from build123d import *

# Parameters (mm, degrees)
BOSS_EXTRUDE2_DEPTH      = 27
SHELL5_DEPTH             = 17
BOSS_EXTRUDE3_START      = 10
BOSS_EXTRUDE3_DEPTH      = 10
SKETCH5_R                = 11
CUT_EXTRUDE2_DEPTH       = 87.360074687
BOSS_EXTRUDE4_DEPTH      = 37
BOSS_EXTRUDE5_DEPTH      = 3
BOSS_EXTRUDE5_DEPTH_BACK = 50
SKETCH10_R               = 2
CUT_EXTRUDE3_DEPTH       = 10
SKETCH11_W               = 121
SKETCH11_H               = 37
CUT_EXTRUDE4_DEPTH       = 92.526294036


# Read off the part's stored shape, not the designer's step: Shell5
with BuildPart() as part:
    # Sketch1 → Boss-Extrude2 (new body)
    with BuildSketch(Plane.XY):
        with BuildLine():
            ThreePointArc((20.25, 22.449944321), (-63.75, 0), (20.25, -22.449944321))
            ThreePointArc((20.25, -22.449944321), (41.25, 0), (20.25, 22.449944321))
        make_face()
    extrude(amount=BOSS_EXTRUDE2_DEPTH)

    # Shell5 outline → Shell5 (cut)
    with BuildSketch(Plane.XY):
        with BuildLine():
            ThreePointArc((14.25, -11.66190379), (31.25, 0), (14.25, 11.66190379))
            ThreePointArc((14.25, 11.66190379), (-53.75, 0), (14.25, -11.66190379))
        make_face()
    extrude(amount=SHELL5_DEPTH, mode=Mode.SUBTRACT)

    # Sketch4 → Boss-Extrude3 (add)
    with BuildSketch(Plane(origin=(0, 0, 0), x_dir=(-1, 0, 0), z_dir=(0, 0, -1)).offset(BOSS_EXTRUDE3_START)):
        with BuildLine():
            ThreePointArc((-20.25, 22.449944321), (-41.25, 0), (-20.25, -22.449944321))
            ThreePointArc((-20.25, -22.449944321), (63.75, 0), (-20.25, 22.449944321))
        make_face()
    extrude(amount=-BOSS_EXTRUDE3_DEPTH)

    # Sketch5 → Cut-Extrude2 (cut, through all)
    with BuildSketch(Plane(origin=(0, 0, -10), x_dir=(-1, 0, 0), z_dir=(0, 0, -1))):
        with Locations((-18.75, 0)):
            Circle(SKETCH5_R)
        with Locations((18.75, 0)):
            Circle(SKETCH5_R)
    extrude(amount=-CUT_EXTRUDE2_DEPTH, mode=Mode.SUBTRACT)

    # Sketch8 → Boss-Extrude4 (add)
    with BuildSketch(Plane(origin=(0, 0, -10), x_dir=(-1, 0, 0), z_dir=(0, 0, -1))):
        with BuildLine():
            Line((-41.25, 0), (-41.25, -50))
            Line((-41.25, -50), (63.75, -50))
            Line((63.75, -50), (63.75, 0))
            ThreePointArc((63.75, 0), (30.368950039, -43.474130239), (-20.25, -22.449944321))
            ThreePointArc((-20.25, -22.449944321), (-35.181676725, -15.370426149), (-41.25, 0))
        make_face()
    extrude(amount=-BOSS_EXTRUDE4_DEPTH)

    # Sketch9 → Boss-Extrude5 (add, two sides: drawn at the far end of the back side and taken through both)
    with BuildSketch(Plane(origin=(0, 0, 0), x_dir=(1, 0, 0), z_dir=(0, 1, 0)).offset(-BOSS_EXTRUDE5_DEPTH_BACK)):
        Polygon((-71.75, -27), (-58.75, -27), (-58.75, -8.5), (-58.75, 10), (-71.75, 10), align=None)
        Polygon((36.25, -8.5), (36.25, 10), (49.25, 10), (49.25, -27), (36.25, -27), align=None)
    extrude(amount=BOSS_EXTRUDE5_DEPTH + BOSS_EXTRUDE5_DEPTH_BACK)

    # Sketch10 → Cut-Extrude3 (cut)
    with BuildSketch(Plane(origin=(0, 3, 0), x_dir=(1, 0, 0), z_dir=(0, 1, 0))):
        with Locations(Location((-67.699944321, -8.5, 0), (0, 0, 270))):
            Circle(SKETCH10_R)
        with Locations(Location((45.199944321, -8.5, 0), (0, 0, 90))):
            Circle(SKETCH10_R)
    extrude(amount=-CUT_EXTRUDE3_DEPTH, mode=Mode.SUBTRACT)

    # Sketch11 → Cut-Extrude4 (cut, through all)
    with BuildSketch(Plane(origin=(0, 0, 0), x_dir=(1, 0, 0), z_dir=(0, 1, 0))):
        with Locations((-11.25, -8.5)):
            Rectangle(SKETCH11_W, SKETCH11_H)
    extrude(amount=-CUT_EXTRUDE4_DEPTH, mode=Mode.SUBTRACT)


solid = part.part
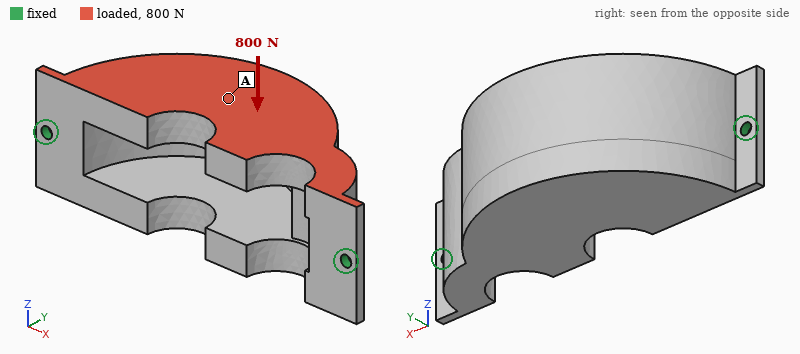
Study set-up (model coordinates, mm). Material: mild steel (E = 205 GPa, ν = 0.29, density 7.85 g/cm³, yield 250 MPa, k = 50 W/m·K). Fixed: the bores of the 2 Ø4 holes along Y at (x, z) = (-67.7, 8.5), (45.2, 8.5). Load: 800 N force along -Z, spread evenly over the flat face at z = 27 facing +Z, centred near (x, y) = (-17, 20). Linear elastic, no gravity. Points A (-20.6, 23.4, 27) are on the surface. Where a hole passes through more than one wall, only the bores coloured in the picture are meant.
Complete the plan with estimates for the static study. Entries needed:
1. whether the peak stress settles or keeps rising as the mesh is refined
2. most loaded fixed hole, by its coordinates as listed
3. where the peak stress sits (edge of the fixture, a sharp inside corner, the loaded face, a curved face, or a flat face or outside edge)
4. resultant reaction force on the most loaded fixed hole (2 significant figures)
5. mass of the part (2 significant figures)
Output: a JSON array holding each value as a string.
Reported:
["keeps rising", "(-67.7, 8.5)", "edge of the fixture", "430 N", "680 g"]
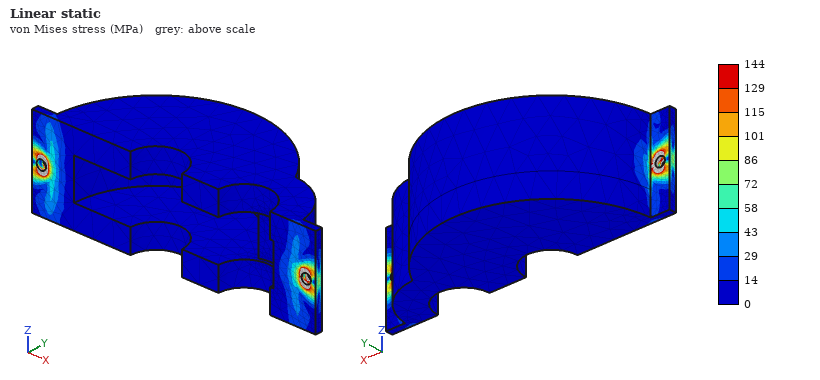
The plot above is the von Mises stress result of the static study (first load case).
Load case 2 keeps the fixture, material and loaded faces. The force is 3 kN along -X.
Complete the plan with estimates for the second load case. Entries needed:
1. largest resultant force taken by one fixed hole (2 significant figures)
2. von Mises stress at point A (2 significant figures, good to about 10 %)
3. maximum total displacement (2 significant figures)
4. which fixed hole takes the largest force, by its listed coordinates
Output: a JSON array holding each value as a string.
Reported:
["1.9 kN", "10 MPa", "7.6 µm", "(-67.7, 8.5)"]
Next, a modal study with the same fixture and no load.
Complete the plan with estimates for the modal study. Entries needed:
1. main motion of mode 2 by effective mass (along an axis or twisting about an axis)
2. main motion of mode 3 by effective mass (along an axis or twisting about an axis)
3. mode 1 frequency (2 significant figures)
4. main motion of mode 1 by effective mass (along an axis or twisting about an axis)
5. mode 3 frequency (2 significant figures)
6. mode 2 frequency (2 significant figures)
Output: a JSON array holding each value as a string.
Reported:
["along Y", "along X", "640 Hz", "along Z", "5600 Hz", "3900 Hz"]
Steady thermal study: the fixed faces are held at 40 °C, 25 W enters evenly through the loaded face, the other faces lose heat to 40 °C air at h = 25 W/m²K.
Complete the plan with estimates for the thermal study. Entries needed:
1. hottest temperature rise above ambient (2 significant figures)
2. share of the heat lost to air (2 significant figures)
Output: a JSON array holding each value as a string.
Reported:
["32 K", "42 %"]
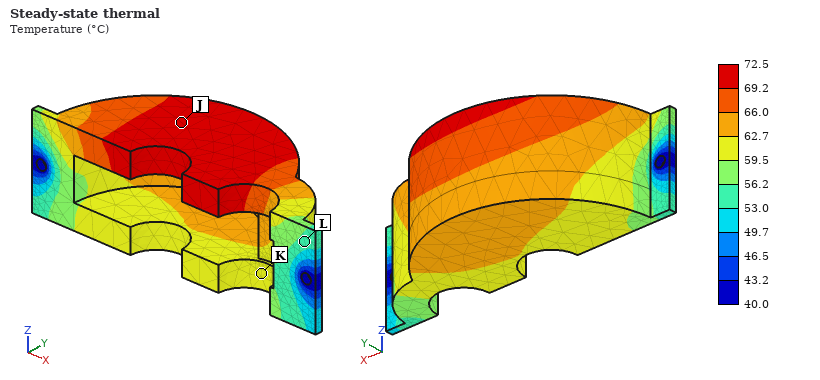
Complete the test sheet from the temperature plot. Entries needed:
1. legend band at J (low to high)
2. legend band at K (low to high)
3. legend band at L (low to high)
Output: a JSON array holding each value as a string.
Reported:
["69.2 to 72.5 °C", "59.5 to 62.7 °C", "53.0 to 56.2 °C"]
